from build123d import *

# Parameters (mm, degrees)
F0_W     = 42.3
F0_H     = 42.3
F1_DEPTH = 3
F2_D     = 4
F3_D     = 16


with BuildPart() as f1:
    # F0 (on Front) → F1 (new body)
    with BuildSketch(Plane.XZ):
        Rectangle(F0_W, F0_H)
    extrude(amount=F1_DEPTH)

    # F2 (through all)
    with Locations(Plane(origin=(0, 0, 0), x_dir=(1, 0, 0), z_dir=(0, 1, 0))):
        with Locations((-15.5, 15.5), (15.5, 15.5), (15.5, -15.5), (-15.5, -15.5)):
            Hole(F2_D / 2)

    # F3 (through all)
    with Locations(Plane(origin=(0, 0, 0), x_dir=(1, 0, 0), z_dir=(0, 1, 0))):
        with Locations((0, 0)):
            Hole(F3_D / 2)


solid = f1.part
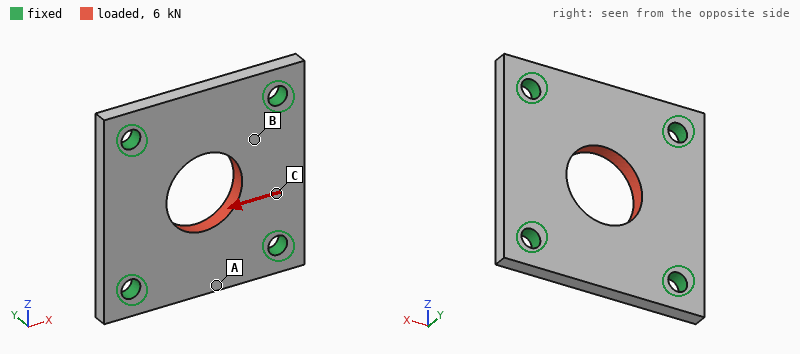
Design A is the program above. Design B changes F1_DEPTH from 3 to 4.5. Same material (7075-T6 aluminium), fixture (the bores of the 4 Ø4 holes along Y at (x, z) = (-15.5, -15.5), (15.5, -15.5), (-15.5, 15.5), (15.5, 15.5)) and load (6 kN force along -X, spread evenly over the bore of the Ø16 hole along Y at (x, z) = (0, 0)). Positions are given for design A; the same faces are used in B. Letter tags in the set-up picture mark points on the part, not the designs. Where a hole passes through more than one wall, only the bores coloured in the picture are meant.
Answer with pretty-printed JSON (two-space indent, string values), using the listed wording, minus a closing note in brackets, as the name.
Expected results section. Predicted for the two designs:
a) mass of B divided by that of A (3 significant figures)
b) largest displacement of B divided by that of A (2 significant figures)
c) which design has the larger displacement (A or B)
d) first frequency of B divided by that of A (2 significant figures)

{
  "mass of B divided by that of A": "1.50",
  "largest displacement of B divided by that of A": "0.67",
  "which design has the larger displacement": "A",
  "first frequency of B divided by that of A": "1.4"
}
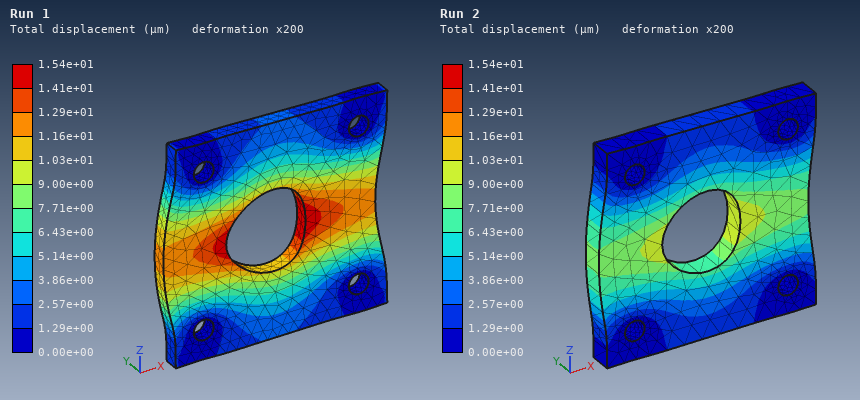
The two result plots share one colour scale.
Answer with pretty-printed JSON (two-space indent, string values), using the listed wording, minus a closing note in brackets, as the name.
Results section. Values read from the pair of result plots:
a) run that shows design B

{
  "run that shows design B": "Run 2"
}
